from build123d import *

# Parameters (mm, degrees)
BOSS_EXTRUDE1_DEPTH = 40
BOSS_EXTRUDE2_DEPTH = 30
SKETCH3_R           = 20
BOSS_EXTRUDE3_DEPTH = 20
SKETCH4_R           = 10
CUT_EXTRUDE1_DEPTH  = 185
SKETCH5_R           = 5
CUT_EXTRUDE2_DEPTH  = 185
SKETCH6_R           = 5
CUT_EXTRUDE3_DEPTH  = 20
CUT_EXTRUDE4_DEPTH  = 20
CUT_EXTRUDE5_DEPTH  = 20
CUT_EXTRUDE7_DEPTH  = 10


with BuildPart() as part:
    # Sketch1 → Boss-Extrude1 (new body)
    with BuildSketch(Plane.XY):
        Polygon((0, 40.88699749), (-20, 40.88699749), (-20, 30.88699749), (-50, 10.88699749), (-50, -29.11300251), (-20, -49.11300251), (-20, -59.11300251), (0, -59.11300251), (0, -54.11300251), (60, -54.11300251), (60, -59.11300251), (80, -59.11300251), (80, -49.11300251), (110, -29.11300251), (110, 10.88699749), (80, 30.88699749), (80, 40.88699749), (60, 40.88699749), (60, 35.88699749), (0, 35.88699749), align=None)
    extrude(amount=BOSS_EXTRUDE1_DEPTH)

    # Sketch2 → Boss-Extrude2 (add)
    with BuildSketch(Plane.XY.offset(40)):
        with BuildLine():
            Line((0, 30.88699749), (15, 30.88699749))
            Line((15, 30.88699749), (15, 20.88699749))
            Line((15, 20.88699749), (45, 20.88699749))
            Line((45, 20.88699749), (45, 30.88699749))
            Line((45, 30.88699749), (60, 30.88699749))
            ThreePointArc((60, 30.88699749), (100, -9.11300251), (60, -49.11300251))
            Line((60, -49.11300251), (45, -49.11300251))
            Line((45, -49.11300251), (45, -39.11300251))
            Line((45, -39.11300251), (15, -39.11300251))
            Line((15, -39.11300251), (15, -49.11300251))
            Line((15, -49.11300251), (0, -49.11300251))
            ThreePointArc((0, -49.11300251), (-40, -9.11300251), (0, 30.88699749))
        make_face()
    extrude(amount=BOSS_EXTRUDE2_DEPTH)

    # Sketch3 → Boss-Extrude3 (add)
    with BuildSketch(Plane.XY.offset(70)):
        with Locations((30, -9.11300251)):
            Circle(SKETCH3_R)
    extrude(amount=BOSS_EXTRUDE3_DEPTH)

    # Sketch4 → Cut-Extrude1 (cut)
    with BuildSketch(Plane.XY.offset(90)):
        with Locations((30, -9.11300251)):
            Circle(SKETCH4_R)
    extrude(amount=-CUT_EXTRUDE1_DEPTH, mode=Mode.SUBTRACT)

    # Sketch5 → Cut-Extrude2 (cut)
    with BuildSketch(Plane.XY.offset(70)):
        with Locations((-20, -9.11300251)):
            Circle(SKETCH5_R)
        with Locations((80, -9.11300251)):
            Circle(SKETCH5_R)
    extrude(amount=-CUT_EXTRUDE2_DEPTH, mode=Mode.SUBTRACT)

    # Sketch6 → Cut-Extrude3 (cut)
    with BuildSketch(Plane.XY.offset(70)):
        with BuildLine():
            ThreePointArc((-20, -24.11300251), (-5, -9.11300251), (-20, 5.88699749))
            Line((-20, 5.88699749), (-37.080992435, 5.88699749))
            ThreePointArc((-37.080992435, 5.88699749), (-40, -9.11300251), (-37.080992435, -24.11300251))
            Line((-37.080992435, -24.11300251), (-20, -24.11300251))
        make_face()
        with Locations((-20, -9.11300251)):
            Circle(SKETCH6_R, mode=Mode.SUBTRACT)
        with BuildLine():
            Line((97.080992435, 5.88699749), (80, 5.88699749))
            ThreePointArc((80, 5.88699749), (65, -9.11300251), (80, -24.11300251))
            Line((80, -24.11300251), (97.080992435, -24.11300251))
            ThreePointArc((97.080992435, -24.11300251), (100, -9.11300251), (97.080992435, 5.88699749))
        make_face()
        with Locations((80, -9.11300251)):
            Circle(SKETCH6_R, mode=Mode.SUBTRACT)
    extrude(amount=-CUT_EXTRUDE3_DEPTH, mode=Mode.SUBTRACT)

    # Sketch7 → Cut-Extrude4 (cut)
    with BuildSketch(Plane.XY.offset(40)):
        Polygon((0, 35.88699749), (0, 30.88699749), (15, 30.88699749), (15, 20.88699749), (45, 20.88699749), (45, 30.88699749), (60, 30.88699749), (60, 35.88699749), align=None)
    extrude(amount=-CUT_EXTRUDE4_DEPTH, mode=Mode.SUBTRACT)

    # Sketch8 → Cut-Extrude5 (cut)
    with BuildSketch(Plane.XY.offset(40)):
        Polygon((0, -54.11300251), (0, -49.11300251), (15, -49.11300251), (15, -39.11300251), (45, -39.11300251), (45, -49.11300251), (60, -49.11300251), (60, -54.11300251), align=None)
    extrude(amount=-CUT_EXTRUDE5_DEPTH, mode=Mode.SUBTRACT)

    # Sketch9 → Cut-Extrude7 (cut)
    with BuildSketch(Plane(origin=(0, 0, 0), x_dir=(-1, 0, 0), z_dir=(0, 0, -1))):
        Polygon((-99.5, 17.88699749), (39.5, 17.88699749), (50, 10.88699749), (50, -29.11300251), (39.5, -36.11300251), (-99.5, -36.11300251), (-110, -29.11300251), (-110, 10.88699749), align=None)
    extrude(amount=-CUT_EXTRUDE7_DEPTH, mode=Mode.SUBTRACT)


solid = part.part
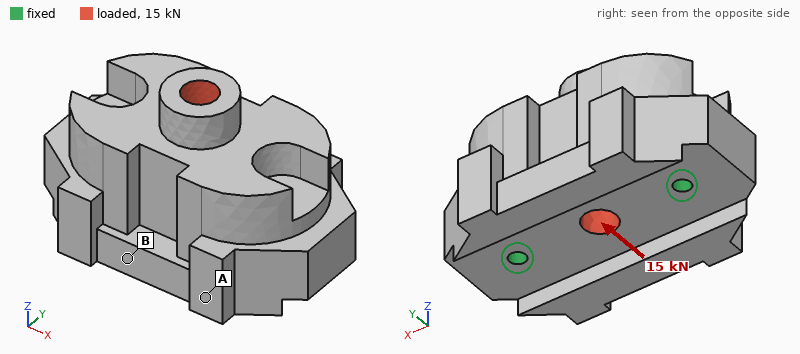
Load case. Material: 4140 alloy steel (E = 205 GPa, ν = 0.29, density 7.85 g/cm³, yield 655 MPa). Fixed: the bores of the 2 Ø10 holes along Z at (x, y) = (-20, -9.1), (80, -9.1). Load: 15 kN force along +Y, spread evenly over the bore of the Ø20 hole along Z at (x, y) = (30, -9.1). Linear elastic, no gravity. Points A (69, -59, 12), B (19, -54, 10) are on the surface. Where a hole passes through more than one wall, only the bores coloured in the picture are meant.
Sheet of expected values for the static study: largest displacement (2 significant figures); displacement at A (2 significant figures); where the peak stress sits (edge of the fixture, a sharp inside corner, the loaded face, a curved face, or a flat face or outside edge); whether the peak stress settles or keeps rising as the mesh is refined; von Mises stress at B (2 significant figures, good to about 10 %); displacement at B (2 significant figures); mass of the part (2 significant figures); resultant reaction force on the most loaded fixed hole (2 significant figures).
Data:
7.5 µm
2.6 µm
edge of the fixture
keeps rising
5.9 MPa
2.1 µm
5.1 kg
7.5 kN
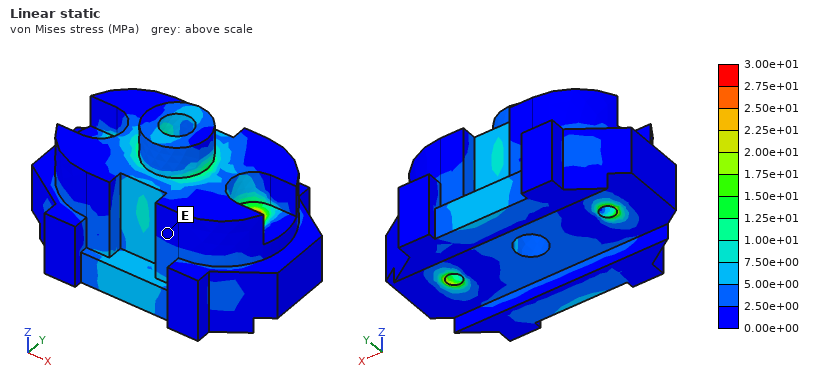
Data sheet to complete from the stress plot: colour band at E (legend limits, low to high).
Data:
0.00e+00 to 2.50e+00 MPa
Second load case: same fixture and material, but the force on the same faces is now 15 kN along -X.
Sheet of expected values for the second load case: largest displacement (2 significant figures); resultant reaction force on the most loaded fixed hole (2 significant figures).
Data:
3.1 µm
8.0 kN
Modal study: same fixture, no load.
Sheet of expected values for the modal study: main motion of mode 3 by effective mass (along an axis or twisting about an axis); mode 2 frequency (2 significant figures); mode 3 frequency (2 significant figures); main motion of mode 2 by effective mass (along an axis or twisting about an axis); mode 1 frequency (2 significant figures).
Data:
along Y
8100 Hz
9100 Hz
along Z
5400 Hz
